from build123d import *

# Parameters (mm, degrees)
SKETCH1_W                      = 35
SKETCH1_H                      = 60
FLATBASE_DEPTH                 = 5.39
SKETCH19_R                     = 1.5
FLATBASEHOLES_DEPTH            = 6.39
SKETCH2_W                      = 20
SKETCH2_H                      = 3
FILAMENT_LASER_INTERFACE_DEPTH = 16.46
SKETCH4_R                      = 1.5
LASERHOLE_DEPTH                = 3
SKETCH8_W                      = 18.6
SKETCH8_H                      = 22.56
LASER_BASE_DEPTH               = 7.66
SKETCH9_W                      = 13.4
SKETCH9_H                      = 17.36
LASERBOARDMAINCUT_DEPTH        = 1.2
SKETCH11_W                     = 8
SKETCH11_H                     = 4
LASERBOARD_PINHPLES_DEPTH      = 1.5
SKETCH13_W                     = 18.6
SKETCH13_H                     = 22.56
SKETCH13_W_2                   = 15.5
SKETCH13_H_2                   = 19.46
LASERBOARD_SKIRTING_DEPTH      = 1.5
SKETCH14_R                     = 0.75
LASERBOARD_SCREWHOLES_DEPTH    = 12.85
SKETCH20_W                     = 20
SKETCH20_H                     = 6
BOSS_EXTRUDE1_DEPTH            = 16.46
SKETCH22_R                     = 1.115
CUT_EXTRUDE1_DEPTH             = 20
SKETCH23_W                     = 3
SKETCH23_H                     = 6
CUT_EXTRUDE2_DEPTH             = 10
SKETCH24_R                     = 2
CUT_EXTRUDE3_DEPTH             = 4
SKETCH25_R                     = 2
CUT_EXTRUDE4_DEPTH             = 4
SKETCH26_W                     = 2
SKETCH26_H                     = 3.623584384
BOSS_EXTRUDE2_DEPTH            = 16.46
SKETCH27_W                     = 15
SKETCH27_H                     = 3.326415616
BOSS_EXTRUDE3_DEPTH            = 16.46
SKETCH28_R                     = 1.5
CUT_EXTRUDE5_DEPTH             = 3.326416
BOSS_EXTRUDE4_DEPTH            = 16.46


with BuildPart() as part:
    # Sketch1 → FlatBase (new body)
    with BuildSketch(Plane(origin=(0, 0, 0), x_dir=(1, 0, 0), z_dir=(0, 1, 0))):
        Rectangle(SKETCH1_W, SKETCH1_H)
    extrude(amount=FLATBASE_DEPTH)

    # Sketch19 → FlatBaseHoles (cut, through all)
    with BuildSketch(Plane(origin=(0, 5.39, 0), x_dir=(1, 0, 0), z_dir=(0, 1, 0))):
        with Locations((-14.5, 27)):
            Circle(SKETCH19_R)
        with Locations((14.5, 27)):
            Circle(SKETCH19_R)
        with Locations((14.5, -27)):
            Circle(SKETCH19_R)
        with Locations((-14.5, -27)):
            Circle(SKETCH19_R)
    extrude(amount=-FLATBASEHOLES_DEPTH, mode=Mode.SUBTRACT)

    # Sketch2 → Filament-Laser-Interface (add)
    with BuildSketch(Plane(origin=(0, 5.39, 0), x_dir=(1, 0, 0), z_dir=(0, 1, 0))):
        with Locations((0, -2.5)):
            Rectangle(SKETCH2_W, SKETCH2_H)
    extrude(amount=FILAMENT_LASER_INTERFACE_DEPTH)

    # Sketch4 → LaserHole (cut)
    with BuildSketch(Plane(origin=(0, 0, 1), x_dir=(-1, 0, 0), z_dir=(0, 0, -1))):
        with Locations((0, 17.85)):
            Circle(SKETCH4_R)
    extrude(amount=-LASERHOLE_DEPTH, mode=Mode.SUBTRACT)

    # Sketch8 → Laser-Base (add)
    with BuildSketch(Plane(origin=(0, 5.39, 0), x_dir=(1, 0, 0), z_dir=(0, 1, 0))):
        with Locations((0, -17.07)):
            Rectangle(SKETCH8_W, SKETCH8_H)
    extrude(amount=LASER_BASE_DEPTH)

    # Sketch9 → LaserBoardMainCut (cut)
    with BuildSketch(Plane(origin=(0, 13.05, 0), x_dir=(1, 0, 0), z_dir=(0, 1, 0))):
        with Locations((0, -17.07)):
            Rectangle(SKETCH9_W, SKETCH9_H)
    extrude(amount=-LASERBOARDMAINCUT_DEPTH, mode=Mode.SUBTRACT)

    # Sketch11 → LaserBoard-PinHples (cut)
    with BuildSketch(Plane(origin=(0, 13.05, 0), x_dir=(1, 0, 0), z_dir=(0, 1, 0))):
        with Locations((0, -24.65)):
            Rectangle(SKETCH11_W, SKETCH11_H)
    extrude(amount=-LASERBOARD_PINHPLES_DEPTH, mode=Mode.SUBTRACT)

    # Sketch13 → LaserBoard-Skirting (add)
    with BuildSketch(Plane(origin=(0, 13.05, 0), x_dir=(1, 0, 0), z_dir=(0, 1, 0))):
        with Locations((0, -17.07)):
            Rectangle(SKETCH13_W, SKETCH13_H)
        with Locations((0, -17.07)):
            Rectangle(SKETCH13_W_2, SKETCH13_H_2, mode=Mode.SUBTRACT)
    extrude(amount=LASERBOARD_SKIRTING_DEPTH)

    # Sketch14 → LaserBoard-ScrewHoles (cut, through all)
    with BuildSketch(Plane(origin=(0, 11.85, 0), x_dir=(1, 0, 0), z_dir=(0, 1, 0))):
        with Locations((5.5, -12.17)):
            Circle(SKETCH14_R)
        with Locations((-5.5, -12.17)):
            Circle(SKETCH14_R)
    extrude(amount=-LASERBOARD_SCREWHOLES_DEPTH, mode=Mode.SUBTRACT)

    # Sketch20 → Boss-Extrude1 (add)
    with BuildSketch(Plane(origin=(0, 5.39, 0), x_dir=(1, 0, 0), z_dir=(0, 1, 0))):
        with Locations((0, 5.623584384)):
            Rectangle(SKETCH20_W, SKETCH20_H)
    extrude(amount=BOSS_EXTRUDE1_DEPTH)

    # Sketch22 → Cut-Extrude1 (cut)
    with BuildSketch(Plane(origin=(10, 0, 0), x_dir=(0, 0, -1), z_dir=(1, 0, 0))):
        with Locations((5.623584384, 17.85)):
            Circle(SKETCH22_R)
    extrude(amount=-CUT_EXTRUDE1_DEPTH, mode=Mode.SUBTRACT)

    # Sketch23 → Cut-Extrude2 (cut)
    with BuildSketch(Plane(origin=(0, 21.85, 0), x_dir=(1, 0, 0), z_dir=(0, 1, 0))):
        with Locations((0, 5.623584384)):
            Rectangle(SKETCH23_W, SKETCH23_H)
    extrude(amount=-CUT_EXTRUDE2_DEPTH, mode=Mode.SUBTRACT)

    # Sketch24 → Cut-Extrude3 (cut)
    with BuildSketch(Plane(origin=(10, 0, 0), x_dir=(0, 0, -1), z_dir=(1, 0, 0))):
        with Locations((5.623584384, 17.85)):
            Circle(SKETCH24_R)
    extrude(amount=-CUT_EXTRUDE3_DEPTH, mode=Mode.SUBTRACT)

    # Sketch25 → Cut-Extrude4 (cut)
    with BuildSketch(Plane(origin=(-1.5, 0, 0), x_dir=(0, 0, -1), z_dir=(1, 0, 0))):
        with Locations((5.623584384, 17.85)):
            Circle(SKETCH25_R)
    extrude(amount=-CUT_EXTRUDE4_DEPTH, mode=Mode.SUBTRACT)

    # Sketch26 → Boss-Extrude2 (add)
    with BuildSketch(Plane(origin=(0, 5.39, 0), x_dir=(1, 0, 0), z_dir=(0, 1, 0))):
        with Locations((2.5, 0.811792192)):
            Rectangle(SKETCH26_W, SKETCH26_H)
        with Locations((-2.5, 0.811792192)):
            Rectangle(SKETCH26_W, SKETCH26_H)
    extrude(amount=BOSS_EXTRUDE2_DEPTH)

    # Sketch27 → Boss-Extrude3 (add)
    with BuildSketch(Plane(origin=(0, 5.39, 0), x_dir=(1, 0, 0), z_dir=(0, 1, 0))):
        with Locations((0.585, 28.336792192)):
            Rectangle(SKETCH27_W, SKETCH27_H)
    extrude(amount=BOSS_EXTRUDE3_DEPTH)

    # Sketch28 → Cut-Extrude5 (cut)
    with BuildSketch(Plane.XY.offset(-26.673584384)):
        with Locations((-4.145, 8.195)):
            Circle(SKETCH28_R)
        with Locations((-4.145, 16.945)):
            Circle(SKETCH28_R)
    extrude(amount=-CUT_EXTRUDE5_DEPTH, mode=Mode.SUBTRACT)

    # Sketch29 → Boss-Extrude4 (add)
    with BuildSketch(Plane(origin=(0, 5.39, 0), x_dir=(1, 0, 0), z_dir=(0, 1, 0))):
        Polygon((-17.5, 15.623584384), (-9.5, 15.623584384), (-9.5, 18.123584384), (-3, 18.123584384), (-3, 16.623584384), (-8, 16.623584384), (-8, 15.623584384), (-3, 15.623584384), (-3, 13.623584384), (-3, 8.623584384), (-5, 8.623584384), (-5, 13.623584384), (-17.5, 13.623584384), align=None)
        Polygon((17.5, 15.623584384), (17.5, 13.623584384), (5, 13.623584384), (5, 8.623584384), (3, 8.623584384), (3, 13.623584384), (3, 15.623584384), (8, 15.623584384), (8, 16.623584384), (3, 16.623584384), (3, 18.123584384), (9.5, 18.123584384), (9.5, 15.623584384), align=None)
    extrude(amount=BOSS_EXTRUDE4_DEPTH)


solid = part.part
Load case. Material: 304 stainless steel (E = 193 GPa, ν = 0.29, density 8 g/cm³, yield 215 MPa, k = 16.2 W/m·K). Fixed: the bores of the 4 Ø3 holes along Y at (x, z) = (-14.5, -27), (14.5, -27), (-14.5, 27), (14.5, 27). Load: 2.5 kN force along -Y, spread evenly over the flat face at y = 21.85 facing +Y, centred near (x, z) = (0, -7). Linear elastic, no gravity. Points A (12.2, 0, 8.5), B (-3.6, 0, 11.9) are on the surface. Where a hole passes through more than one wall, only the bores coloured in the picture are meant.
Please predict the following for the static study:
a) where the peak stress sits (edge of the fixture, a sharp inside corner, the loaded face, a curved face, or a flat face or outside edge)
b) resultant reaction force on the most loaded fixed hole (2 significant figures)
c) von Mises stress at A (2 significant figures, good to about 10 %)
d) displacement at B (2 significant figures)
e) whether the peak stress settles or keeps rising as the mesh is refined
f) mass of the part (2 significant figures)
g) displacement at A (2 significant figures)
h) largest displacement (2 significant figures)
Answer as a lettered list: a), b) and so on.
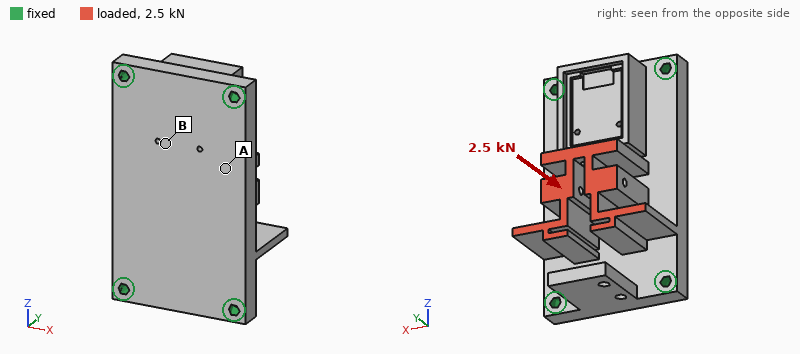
a) edge of the fixture
b) 820 N
c) 28 MPa
d) 13 µm
e) keeps rising
f) 160 g
g) 15 µm
h) 21 µm
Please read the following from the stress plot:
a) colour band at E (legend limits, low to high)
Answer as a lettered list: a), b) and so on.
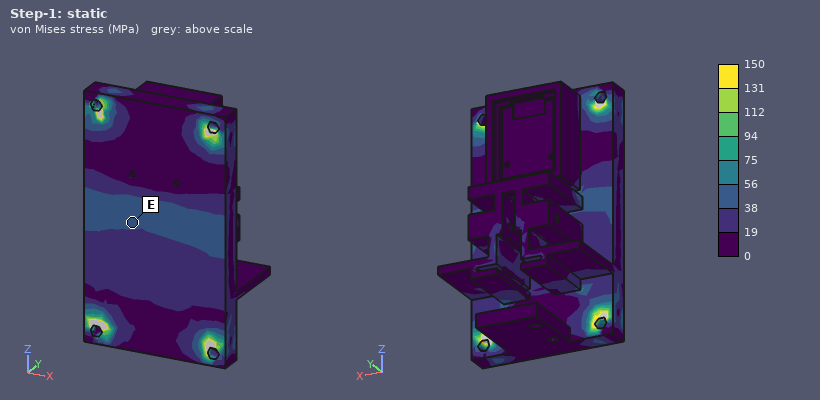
a) 38 to 56 MPa
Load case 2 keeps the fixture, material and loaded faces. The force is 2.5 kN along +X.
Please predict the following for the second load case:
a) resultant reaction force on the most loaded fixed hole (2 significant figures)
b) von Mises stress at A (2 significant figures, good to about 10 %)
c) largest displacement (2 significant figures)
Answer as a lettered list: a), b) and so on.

a) 1.3 kN
b) 22 MPa
c) 36 µm
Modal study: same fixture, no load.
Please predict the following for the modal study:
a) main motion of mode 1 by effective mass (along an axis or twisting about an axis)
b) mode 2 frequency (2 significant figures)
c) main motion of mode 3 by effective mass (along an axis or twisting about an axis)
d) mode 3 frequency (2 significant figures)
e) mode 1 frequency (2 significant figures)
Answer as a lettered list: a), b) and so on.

a) along Y
b) 7400 Hz
c) along X
d) 9800 Hz
e) 5900 Hz
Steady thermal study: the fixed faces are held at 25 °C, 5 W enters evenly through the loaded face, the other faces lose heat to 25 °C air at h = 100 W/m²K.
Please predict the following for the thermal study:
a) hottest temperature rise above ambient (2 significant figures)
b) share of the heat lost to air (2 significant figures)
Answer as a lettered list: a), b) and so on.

a) 18 K
b) 85 %
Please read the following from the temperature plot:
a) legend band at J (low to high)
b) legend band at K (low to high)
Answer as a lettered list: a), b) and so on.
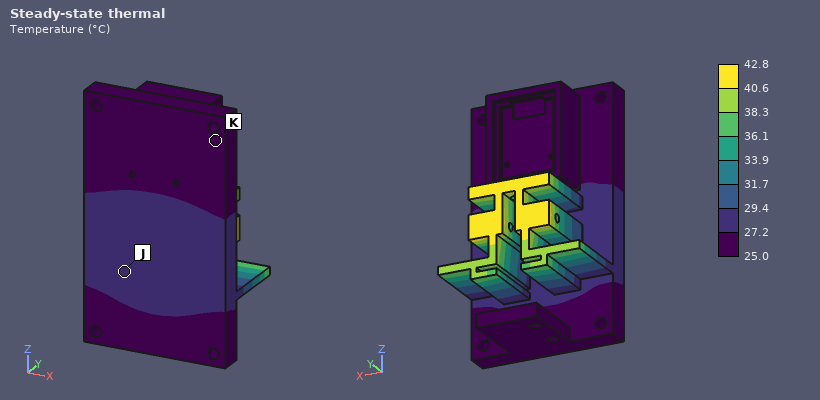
a) 27.2 to 29.4 °C
b) 25.0 to 27.2 °C
